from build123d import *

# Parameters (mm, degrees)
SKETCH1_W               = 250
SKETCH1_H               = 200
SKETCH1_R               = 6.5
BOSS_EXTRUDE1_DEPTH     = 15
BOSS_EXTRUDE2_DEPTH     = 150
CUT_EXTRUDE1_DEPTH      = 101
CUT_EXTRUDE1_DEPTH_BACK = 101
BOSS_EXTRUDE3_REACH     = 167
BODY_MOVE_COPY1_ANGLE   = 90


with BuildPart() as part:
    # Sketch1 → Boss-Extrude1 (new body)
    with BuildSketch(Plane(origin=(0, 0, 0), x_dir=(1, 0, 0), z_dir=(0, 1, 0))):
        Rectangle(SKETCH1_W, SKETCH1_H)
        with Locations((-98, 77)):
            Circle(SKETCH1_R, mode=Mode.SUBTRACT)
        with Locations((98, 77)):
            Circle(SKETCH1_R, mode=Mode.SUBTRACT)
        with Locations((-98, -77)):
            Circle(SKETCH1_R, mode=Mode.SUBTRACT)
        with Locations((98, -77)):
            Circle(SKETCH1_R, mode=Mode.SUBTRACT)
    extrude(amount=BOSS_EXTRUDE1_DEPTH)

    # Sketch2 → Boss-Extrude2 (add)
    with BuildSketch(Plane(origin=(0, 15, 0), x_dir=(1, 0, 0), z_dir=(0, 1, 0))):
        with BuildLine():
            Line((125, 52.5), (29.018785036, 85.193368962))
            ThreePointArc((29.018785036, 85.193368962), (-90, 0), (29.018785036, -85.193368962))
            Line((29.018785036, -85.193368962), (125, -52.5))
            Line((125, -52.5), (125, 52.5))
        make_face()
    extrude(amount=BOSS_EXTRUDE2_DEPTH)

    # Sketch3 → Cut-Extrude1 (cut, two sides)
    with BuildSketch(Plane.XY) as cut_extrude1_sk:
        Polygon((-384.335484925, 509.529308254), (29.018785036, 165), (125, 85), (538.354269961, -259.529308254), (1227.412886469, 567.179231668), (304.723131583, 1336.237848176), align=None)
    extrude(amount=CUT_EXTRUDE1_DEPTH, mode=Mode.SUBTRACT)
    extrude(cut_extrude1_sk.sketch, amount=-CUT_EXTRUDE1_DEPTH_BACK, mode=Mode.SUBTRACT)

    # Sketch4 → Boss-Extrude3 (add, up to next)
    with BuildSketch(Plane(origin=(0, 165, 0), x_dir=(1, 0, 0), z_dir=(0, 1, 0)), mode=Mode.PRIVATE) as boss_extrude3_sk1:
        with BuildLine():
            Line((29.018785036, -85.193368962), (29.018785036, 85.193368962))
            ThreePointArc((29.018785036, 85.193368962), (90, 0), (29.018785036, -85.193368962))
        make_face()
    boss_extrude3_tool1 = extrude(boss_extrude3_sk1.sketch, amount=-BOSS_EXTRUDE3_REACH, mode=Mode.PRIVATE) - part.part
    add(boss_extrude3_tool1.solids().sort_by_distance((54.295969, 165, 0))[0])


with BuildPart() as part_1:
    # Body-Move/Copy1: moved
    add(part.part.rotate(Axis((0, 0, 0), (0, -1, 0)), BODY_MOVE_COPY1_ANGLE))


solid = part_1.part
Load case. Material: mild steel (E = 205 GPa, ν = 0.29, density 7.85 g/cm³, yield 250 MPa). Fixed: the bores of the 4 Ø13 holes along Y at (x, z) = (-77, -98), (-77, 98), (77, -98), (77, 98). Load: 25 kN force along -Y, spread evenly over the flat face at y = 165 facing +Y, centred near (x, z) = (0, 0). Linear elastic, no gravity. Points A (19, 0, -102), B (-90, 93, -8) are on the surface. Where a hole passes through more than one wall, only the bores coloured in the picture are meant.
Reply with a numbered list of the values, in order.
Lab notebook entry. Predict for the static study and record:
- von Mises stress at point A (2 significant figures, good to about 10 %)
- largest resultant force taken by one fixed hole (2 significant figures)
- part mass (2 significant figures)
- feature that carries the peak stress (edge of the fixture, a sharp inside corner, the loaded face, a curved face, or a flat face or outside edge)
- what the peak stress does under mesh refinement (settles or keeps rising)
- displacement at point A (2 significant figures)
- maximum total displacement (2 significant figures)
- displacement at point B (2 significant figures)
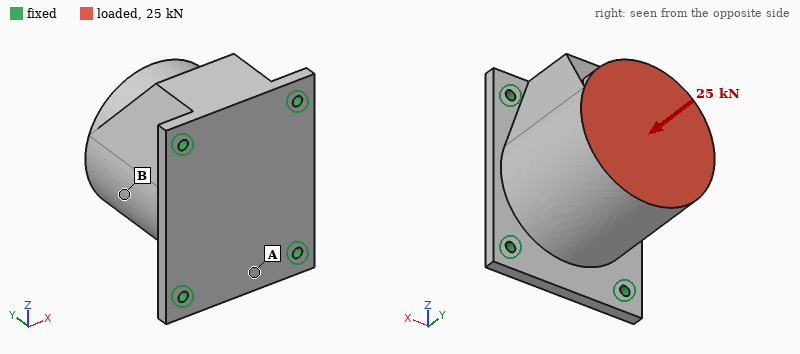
1. 12 MPa
2. 6.9 kN
3. 40 kg
4. edge of the fixture
5. keeps rising
6. 14 µm
7. 20 µm
8. 13 µm
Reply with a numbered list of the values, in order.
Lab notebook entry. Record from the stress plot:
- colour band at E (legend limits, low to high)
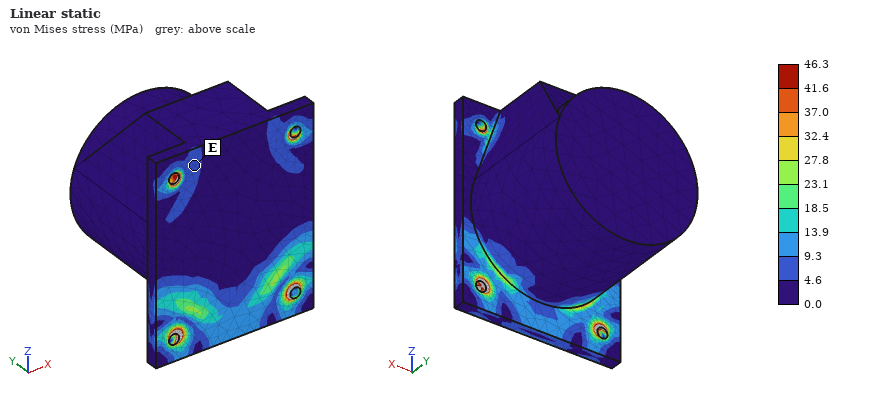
1. 4.6 to 9.3 MPa
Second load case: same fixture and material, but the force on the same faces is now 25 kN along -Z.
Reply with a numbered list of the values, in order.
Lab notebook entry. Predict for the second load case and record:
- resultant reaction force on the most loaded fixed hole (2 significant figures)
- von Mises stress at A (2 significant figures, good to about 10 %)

1. 13 kN
2. 22 MPa
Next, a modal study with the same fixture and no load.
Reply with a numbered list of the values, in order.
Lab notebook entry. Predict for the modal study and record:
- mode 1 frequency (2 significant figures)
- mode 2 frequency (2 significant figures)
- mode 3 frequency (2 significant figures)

1. 1000 Hz
2. 1000 Hz
3. 1700 Hz
